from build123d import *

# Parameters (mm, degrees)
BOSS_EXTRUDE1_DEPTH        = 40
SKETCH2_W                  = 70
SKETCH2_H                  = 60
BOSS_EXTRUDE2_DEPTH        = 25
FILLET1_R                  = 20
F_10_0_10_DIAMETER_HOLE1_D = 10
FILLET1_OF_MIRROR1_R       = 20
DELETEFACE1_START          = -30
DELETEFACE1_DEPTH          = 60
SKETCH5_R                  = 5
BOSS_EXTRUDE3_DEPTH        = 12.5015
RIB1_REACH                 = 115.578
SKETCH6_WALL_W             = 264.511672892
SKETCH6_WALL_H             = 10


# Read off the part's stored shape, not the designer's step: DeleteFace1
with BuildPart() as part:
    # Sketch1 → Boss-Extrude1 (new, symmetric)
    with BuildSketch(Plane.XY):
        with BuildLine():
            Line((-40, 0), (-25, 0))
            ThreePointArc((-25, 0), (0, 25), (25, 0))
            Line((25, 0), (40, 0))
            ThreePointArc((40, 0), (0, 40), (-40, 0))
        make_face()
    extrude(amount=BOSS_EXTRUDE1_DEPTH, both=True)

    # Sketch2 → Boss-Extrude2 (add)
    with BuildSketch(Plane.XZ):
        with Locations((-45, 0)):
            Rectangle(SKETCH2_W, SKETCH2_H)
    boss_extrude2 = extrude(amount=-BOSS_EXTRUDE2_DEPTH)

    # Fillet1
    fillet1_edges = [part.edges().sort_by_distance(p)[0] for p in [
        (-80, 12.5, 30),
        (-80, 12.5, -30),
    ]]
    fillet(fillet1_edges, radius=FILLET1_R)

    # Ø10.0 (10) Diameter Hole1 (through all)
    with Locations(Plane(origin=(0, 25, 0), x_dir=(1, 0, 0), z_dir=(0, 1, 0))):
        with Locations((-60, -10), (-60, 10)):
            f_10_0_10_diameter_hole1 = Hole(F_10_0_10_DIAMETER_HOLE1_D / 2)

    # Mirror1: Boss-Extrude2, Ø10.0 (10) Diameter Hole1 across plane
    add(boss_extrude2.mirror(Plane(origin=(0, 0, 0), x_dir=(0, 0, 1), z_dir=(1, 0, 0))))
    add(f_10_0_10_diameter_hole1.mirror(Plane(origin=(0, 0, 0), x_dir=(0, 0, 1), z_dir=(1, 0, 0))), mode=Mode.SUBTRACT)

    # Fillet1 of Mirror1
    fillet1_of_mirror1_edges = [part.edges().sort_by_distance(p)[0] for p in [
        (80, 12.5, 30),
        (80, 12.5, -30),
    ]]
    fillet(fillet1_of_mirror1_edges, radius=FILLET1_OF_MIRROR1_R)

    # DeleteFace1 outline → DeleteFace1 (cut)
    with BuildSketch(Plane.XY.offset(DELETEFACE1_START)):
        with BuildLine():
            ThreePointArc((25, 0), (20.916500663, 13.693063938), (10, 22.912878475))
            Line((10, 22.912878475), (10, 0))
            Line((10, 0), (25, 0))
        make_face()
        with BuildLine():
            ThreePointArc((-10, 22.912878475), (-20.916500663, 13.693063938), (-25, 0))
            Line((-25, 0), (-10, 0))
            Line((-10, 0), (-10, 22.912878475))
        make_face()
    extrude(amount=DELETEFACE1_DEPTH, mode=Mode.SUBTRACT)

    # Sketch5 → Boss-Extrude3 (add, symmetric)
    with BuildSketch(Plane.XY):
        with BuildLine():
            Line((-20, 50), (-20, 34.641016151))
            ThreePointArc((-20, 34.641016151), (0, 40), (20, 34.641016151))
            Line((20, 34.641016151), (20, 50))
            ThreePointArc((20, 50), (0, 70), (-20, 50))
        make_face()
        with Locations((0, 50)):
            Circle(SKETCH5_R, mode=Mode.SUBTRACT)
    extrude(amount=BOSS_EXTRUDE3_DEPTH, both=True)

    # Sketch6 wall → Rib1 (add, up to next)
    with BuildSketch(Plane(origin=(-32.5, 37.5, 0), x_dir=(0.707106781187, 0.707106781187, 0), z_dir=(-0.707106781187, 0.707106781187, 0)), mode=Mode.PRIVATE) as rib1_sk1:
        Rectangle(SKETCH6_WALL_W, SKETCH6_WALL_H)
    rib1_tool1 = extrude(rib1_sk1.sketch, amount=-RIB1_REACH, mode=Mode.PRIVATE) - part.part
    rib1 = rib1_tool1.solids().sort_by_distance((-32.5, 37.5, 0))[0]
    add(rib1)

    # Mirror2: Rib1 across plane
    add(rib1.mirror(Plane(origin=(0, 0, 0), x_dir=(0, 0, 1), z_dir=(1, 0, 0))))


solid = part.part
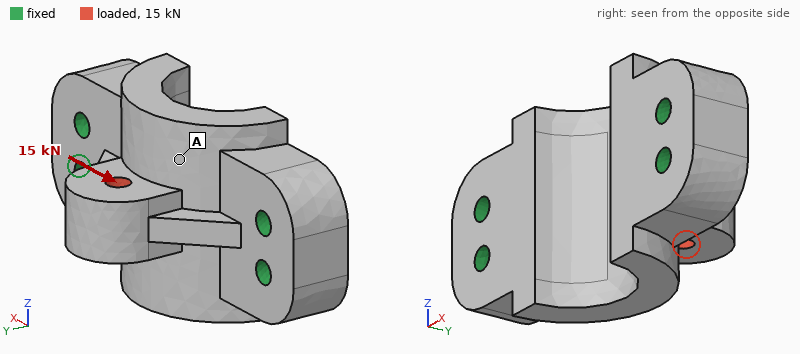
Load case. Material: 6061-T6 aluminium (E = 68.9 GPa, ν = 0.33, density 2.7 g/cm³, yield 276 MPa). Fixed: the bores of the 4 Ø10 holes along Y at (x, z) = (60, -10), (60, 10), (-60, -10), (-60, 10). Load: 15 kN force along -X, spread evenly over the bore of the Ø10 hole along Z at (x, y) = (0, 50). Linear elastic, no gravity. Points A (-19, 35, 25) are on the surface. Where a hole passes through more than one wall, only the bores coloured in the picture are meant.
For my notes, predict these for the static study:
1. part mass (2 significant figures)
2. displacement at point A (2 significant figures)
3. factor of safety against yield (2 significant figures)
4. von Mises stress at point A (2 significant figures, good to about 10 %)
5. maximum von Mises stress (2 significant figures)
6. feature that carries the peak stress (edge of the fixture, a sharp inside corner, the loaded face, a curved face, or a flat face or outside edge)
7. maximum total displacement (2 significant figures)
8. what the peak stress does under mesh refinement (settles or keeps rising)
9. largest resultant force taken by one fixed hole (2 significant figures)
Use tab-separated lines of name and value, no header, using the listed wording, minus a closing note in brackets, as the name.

part mass	720 g
displacement at point A	8.1 µm
factor of safety against yield	5.6
von Mises stress at point A	7.0 MPa
maximum von Mises stress	49 MPa
feature that carries the peak stress	the loaded face
maximum total displacement	34 µm
what the peak stress does under mesh refinement	settles
largest resultant force taken by one fixed hole	4.9 kN
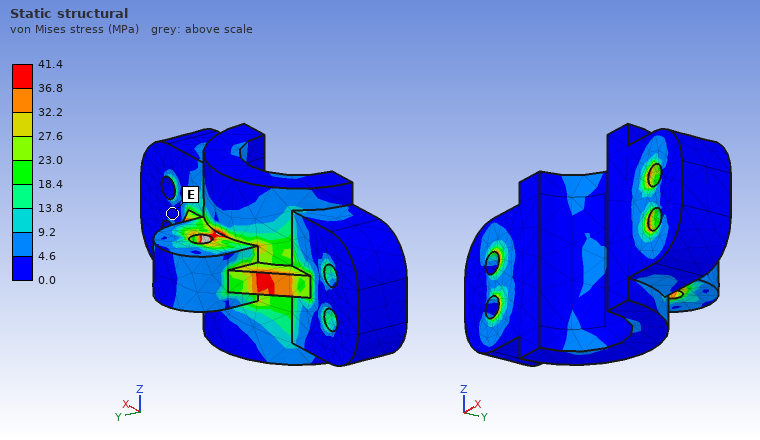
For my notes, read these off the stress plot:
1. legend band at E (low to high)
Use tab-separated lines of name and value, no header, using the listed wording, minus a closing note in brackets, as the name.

legend band at E	0.0 to 4.6 MPa
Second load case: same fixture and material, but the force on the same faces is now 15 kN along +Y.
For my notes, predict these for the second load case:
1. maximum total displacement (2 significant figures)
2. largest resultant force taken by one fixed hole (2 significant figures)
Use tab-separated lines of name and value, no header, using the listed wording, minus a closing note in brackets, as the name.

maximum total displacement	27 µm
largest resultant force taken by one fixed hole	5.5 kN
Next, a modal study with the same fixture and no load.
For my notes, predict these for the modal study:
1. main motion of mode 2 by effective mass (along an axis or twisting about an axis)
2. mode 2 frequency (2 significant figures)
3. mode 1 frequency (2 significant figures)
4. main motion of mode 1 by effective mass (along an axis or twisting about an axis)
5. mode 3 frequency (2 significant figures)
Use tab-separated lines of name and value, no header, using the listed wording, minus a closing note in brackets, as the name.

main motion of mode 2 by effective mass	along Y
mode 2 frequency	7500 Hz
mode 1 frequency	4800 Hz
main motion of mode 1 by effective mass	along Z
mode 3 frequency	10 kHz
